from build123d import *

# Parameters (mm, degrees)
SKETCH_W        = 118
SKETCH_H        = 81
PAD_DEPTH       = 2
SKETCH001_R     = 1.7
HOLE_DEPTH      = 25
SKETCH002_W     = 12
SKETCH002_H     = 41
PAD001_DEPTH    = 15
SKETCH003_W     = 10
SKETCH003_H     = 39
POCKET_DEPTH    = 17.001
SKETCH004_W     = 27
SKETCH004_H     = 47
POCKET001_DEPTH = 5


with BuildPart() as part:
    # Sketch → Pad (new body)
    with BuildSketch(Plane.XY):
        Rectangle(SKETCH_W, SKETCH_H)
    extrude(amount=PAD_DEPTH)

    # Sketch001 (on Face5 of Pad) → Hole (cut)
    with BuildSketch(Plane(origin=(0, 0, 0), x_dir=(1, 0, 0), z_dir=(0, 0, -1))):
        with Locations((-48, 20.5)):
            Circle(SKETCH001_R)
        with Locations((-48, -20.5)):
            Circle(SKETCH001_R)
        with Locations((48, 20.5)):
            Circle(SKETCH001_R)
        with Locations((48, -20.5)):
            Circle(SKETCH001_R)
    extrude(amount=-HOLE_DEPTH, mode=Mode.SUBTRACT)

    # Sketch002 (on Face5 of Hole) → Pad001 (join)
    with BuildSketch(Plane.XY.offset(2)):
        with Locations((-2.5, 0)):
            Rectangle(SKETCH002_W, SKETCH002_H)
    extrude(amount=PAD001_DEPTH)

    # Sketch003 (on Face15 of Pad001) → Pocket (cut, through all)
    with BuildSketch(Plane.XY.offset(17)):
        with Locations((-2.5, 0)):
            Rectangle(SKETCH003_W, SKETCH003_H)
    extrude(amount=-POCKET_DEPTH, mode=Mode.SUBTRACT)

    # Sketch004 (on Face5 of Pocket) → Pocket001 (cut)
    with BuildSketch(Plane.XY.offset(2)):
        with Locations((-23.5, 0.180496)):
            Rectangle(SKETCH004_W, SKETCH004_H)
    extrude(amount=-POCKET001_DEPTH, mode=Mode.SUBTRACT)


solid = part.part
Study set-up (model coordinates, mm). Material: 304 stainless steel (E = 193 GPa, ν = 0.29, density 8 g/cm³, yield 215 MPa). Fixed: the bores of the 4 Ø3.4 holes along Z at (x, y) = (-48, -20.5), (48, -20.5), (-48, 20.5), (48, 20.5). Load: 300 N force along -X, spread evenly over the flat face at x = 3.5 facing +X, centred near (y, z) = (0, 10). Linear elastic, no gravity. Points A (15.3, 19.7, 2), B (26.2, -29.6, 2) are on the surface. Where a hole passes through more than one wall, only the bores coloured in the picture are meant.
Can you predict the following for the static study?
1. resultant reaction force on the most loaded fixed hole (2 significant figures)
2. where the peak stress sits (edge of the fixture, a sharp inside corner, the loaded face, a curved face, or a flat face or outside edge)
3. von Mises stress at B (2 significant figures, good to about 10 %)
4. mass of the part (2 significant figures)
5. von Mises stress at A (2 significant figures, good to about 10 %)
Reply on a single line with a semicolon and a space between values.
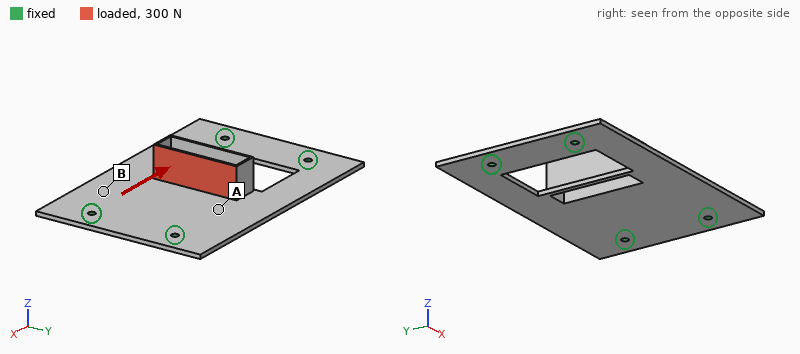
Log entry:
130 N; a flat face or outside edge; 9.2 MPa; 140 g; 16 MPa
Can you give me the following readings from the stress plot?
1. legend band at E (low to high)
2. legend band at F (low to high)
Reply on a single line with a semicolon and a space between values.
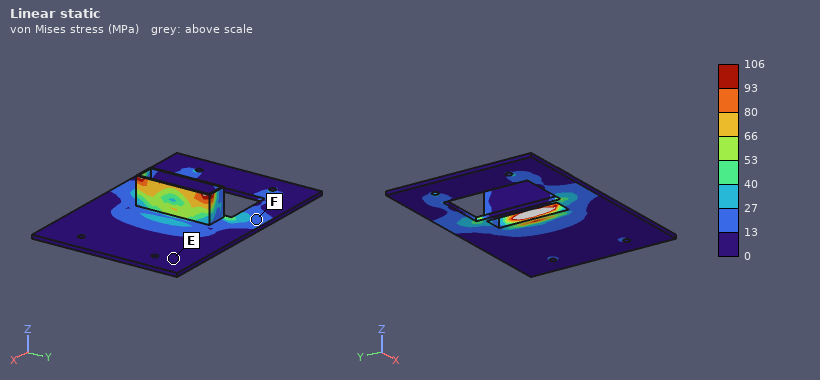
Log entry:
0 to 13 MPa; 13 to 27 MPa
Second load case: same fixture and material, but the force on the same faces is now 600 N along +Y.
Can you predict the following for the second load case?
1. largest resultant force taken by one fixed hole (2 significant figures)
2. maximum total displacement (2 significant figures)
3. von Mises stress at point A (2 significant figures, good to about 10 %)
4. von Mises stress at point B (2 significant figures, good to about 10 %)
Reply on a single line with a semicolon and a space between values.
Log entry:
370 N; 0.13 mm; 31 MPa; 17 MPa
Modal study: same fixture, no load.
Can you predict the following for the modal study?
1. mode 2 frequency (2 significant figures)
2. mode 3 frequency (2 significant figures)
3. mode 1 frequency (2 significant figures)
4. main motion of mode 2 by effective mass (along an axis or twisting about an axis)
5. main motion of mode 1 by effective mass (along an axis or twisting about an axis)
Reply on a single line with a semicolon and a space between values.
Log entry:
1100 Hz; 2300 Hz; 850 Hz; twisting about X; along Z
